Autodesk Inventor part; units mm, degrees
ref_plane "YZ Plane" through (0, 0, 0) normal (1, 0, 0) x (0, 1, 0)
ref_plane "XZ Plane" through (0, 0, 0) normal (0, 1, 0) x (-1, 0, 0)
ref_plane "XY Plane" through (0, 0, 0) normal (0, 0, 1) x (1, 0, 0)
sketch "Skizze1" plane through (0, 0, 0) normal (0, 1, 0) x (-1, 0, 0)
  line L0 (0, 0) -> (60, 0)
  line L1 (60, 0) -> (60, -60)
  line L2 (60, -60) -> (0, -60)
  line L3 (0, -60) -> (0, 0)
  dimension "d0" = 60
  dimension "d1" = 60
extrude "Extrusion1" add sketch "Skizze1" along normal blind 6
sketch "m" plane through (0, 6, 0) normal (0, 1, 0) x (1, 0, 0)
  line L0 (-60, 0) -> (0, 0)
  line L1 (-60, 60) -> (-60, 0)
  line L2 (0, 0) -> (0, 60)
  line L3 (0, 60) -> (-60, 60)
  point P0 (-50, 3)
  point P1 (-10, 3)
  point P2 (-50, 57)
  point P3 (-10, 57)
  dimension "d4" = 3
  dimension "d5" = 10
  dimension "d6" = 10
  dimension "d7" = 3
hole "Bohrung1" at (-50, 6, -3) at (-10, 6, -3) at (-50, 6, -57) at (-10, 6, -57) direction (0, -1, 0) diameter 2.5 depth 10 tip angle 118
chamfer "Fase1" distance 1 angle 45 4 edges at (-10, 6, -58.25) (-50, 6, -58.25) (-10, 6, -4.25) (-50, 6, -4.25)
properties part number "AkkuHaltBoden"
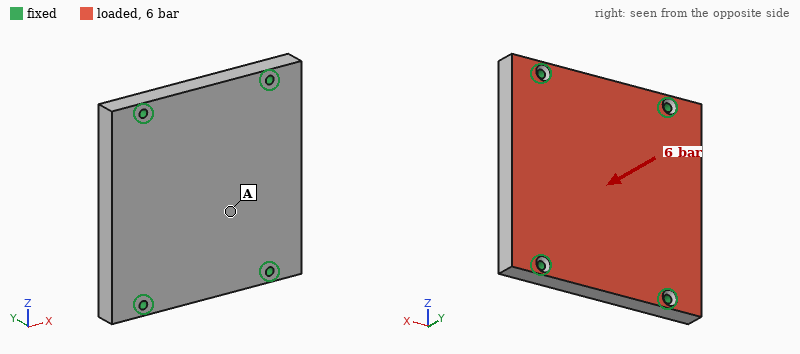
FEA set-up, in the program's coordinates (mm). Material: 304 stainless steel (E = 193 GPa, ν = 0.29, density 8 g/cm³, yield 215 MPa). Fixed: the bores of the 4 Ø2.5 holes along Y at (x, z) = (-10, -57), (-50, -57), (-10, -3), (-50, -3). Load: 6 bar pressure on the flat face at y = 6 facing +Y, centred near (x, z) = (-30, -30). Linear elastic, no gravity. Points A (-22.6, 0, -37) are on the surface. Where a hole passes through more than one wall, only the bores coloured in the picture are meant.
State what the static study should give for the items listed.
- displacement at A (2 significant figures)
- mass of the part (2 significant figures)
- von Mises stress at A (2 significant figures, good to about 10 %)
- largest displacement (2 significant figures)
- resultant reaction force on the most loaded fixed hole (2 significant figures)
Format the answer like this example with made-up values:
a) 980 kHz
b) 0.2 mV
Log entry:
a) 8.5 µm
b) 170 g
c) 13 MPa
d) 9.3 µm
e) 540 N
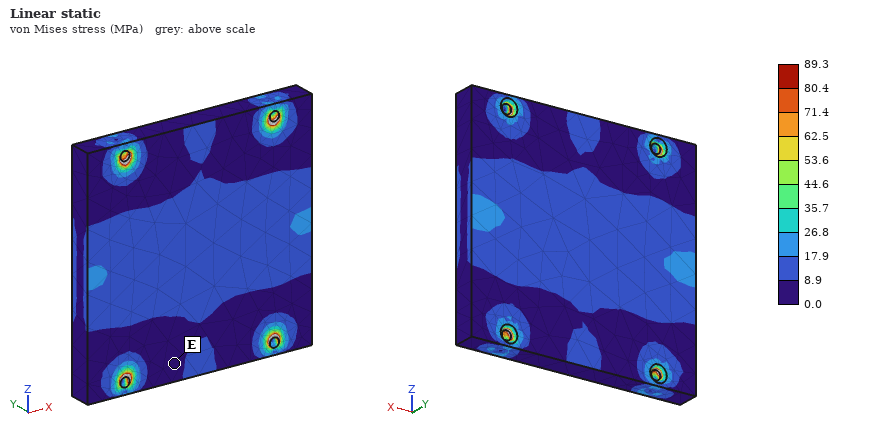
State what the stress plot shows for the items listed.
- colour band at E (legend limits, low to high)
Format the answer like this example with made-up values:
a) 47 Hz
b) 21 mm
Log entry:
a) 0.0 to 8.9 MPa
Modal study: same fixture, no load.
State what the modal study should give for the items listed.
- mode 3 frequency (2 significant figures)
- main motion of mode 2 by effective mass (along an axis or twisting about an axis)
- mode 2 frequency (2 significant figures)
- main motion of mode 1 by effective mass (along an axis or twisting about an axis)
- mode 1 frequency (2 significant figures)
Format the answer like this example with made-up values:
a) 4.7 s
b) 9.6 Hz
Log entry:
a) 12 kHz
b) twisting about Z
c) 9000 Hz
d) along Y
e) 6700 Hz
